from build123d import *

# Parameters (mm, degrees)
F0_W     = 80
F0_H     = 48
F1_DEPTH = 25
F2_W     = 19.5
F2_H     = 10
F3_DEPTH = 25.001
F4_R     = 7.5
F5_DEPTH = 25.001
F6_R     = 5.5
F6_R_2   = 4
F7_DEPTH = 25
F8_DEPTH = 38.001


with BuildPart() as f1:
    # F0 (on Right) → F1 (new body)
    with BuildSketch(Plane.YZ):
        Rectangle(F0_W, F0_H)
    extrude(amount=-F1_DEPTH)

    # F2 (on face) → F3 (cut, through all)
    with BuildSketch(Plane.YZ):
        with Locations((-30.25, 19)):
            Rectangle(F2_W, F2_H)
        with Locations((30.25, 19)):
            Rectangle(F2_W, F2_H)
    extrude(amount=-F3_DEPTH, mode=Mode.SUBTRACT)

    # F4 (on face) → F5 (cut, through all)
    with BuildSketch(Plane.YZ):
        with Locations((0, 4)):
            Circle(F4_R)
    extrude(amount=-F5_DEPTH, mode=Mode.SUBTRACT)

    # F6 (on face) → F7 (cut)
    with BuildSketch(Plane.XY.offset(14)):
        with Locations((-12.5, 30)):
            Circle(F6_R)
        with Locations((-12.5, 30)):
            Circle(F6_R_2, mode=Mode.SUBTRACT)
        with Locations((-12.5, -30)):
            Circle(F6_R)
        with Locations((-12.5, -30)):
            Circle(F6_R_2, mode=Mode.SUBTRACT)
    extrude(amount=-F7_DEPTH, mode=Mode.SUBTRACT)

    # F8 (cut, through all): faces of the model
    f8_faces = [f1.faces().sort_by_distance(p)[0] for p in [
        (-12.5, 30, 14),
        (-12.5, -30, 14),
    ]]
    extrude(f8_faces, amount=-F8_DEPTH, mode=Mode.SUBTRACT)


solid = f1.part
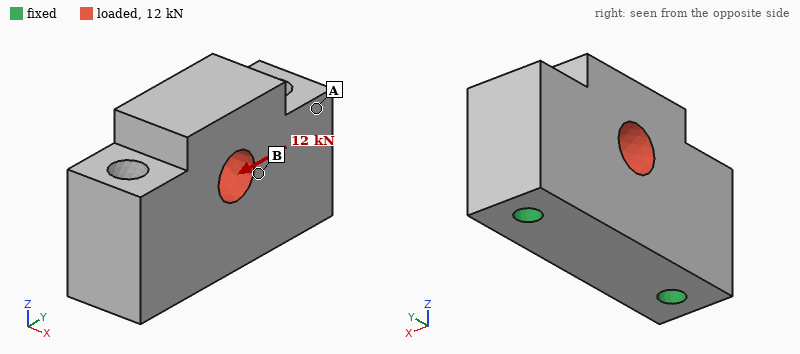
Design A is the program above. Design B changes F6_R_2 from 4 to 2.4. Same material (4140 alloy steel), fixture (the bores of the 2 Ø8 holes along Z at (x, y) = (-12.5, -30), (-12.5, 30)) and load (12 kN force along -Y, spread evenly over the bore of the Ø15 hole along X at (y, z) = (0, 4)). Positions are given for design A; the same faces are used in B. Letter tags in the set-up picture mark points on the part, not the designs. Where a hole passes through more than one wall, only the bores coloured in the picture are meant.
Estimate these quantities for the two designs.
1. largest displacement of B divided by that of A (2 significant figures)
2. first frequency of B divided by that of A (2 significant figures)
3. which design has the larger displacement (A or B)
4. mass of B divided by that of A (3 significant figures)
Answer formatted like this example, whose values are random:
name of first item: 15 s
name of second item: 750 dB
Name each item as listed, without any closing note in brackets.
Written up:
largest displacement of B divided by that of A: 1.2
first frequency of B divided by that of A: 0.80
which design has the larger displacement: B
mass of B divided by that of A: 1.01
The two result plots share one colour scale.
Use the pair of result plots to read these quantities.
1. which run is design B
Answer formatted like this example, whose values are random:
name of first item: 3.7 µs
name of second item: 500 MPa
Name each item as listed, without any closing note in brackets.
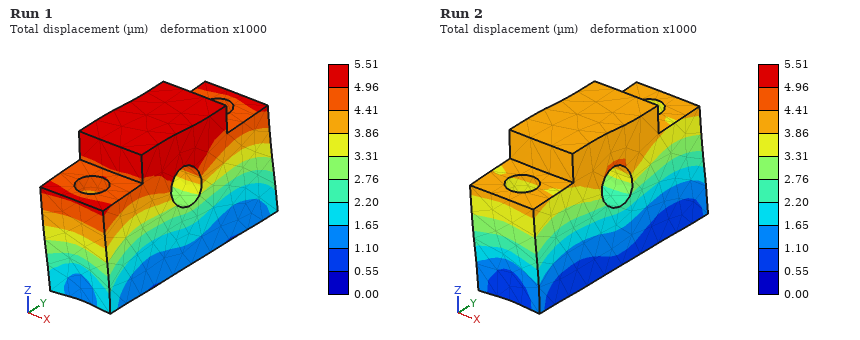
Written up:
which run is design B: Run 1
